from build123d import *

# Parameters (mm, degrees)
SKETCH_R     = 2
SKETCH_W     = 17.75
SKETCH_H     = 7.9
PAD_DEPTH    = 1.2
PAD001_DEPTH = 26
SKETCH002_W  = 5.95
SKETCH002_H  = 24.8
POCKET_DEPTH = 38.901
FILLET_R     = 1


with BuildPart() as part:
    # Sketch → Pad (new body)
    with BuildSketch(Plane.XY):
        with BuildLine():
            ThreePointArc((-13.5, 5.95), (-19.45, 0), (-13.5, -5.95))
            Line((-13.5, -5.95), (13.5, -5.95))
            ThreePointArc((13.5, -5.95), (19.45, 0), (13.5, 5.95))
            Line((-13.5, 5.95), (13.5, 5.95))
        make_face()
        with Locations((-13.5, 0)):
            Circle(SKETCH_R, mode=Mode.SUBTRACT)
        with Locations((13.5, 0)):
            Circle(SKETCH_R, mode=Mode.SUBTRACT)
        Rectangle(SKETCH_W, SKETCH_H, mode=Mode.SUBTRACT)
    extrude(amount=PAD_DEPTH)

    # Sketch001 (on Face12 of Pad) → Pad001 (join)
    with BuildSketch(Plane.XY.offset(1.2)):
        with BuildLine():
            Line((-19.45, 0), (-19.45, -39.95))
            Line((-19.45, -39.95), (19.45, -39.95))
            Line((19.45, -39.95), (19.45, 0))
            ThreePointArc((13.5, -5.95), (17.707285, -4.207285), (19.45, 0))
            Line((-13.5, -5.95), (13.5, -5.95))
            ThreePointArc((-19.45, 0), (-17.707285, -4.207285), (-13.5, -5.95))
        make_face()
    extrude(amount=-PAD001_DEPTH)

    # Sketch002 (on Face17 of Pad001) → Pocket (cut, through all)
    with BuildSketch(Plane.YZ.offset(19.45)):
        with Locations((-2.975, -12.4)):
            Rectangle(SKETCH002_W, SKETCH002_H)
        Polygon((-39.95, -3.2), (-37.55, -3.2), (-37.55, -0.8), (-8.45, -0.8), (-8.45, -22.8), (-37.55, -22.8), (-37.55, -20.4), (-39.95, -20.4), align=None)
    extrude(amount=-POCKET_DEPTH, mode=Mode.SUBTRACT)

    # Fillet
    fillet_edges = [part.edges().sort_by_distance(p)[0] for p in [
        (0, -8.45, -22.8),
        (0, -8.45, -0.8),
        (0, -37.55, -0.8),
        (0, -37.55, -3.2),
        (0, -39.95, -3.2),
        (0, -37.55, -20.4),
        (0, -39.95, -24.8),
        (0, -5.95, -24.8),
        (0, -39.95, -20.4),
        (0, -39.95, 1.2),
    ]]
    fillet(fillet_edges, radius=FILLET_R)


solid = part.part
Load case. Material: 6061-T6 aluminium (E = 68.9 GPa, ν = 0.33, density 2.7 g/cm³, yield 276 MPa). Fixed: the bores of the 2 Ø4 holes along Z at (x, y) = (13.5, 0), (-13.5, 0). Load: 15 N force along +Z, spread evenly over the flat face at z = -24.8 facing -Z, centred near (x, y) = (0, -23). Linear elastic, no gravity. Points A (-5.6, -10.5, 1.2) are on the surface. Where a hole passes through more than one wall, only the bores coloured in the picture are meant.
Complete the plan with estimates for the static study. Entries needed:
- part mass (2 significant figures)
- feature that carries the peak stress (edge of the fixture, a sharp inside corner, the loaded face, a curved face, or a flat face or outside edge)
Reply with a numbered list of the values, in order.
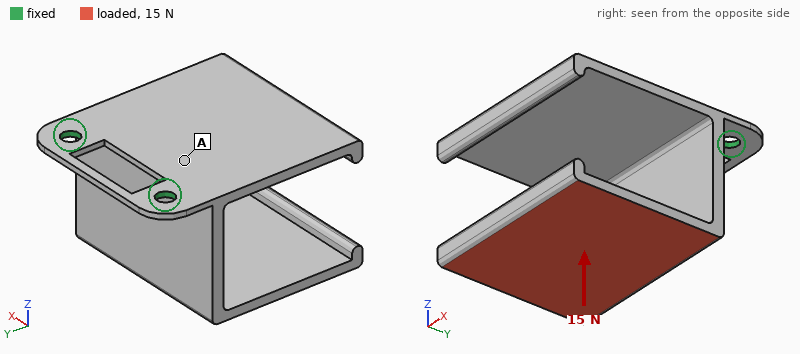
1. 22 g
2. a flat face or outside edge
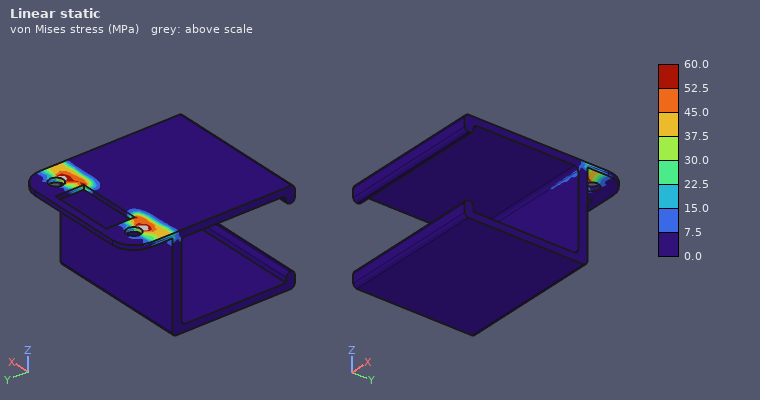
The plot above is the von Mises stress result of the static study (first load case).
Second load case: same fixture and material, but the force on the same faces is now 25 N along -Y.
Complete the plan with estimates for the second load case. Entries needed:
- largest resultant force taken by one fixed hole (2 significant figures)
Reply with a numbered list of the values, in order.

1. 13 N
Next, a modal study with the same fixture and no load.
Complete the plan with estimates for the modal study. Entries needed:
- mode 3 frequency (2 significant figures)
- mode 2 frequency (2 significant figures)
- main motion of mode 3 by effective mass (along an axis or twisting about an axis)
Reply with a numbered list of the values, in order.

1. 1400 Hz
2. 1100 Hz
3. along X
